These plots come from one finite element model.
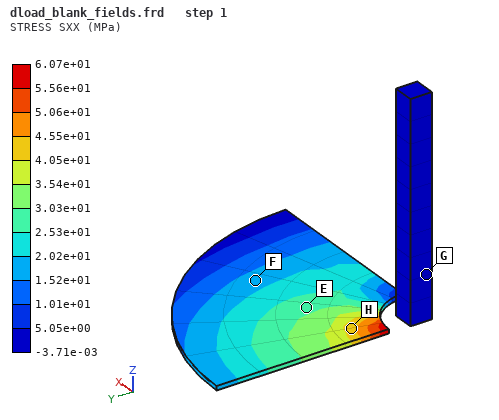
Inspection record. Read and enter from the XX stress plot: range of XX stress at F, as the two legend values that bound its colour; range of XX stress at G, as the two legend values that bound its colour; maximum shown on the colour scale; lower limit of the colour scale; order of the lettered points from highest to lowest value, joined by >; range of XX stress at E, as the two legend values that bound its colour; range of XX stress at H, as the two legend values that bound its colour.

1.52e+01 to 2.02e+01 MPa
-3.71e-03 to 5.05e+00 MPa
6.07e+01 MPa
-3.71e-03 MPa
H > E > F > G
2.53e+01 to 3.03e+01 MPa
4.05e+01 to 4.55e+01 MPa
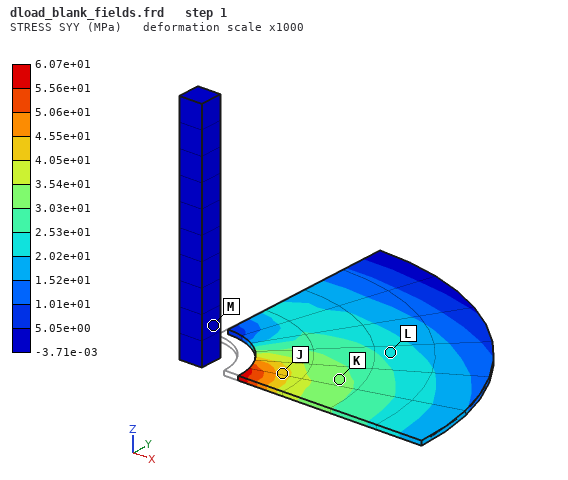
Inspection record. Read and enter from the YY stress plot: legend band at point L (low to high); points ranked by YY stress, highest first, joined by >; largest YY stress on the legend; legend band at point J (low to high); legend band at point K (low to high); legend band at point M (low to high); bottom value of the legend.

2.02e+01 to 2.53e+01 MPa
J > K > L > M
6.07e+01 MPa
4.05e+01 to 4.55e+01 MPa
3.03e+01 to 3.54e+01 MPa
-3.71e-03 to 5.05e+00 MPa
-3.71e-03 MPa
